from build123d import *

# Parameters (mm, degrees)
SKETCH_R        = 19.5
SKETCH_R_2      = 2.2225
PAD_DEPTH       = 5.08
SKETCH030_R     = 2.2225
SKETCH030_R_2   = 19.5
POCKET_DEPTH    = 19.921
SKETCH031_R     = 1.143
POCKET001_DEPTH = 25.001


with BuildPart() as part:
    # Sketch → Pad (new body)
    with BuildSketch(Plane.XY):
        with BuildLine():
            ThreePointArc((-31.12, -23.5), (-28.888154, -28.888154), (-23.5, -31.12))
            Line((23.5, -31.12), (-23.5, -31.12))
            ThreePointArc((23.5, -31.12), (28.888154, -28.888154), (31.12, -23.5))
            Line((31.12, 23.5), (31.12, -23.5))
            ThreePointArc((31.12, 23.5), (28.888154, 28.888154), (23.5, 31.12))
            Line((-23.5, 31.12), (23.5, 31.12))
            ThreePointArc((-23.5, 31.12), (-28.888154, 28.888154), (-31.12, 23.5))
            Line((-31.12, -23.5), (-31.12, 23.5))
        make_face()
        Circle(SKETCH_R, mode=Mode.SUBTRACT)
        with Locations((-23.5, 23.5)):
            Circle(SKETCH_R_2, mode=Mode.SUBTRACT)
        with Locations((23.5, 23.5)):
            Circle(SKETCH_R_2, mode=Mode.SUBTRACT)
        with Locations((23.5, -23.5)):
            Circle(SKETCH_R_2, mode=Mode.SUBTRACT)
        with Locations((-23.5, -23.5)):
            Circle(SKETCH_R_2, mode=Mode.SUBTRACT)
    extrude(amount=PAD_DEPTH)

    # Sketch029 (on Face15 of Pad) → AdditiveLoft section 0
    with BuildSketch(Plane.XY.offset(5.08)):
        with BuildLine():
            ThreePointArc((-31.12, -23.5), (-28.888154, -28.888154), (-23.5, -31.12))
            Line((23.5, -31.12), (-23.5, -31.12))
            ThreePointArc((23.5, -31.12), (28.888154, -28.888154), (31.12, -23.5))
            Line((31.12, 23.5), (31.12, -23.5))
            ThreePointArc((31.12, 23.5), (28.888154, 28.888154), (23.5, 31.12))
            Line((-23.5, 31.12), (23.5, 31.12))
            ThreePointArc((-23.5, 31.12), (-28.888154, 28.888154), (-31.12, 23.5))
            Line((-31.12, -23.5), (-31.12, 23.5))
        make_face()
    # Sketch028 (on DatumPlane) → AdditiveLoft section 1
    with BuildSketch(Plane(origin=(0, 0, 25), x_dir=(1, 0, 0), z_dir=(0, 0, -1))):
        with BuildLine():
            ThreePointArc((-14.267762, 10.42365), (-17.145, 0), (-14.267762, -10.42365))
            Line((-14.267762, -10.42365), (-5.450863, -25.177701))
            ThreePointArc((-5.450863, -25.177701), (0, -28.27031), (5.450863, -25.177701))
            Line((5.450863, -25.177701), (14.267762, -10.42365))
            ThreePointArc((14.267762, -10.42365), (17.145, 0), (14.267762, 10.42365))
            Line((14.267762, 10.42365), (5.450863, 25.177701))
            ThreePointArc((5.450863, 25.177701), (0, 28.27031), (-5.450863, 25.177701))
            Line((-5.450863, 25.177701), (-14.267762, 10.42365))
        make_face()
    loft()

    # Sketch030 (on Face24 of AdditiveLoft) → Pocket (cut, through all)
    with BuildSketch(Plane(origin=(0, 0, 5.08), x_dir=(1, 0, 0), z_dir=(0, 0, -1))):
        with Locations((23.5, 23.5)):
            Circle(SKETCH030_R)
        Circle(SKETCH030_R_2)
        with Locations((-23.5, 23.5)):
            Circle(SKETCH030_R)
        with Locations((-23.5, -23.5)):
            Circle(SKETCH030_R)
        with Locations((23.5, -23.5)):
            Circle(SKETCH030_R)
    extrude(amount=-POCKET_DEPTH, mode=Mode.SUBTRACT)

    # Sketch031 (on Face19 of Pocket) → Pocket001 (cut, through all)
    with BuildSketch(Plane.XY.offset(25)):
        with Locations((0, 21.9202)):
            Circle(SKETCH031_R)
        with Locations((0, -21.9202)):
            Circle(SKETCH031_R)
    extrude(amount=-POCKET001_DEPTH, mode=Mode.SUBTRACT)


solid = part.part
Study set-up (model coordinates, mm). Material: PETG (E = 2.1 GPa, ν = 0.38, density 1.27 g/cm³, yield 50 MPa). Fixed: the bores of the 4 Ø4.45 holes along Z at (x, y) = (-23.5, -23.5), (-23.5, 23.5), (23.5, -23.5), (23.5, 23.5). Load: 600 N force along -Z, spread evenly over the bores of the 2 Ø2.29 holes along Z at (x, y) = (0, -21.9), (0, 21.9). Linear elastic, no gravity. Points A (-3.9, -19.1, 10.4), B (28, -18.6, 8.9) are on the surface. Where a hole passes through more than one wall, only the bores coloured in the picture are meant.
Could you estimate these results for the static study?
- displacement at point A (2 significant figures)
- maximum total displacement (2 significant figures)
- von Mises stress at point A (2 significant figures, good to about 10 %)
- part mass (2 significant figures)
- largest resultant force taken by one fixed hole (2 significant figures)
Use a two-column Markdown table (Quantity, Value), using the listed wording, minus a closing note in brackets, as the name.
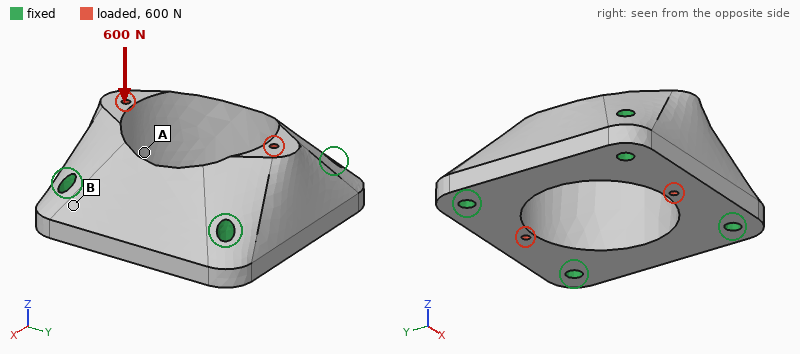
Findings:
| Quantity | Value |
|---|---|
| displacement at point A | 28 µm |
| maximum total displacement | 36 µm |
| von Mises stress at point A | 1.8 MPa |
| part mass | 50 g |
| largest resultant force taken by one fixed hole | 170 N |
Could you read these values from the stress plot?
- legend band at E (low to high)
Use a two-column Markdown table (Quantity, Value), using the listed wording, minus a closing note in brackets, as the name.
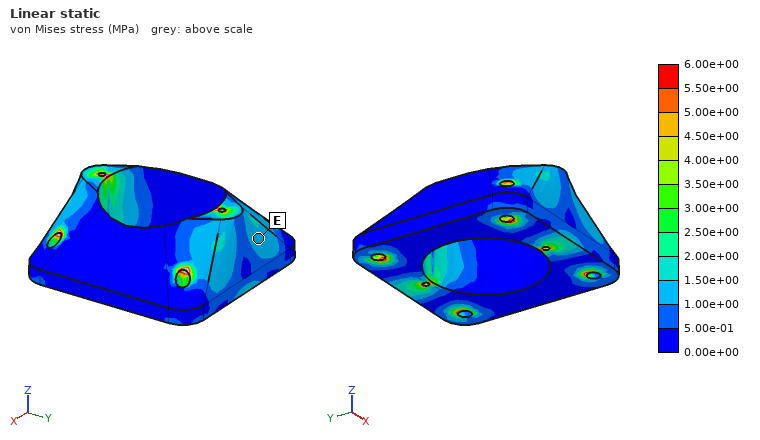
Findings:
| Quantity | Value |
|---|---|
| legend band at E | 1.00e+00 to 1.50e+00 MPa |
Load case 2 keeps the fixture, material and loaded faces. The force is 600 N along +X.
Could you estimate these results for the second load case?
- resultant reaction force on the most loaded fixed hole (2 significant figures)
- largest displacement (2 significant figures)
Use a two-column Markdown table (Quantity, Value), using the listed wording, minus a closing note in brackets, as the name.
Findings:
| Quantity | Value |
|---|---|
| resultant reaction force on the most loaded fixed hole | 150 N |
| largest displacement | 13 µm |
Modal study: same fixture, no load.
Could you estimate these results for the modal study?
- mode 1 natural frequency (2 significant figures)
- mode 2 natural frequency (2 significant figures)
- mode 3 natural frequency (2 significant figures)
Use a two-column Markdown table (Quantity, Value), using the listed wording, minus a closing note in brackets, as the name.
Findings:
| Quantity | Value |
|---|---|
| mode 1 natural frequency | 3500 Hz |
| mode 2 natural frequency | 5000 Hz |
| mode 3 natural frequency | 5100 Hz |
